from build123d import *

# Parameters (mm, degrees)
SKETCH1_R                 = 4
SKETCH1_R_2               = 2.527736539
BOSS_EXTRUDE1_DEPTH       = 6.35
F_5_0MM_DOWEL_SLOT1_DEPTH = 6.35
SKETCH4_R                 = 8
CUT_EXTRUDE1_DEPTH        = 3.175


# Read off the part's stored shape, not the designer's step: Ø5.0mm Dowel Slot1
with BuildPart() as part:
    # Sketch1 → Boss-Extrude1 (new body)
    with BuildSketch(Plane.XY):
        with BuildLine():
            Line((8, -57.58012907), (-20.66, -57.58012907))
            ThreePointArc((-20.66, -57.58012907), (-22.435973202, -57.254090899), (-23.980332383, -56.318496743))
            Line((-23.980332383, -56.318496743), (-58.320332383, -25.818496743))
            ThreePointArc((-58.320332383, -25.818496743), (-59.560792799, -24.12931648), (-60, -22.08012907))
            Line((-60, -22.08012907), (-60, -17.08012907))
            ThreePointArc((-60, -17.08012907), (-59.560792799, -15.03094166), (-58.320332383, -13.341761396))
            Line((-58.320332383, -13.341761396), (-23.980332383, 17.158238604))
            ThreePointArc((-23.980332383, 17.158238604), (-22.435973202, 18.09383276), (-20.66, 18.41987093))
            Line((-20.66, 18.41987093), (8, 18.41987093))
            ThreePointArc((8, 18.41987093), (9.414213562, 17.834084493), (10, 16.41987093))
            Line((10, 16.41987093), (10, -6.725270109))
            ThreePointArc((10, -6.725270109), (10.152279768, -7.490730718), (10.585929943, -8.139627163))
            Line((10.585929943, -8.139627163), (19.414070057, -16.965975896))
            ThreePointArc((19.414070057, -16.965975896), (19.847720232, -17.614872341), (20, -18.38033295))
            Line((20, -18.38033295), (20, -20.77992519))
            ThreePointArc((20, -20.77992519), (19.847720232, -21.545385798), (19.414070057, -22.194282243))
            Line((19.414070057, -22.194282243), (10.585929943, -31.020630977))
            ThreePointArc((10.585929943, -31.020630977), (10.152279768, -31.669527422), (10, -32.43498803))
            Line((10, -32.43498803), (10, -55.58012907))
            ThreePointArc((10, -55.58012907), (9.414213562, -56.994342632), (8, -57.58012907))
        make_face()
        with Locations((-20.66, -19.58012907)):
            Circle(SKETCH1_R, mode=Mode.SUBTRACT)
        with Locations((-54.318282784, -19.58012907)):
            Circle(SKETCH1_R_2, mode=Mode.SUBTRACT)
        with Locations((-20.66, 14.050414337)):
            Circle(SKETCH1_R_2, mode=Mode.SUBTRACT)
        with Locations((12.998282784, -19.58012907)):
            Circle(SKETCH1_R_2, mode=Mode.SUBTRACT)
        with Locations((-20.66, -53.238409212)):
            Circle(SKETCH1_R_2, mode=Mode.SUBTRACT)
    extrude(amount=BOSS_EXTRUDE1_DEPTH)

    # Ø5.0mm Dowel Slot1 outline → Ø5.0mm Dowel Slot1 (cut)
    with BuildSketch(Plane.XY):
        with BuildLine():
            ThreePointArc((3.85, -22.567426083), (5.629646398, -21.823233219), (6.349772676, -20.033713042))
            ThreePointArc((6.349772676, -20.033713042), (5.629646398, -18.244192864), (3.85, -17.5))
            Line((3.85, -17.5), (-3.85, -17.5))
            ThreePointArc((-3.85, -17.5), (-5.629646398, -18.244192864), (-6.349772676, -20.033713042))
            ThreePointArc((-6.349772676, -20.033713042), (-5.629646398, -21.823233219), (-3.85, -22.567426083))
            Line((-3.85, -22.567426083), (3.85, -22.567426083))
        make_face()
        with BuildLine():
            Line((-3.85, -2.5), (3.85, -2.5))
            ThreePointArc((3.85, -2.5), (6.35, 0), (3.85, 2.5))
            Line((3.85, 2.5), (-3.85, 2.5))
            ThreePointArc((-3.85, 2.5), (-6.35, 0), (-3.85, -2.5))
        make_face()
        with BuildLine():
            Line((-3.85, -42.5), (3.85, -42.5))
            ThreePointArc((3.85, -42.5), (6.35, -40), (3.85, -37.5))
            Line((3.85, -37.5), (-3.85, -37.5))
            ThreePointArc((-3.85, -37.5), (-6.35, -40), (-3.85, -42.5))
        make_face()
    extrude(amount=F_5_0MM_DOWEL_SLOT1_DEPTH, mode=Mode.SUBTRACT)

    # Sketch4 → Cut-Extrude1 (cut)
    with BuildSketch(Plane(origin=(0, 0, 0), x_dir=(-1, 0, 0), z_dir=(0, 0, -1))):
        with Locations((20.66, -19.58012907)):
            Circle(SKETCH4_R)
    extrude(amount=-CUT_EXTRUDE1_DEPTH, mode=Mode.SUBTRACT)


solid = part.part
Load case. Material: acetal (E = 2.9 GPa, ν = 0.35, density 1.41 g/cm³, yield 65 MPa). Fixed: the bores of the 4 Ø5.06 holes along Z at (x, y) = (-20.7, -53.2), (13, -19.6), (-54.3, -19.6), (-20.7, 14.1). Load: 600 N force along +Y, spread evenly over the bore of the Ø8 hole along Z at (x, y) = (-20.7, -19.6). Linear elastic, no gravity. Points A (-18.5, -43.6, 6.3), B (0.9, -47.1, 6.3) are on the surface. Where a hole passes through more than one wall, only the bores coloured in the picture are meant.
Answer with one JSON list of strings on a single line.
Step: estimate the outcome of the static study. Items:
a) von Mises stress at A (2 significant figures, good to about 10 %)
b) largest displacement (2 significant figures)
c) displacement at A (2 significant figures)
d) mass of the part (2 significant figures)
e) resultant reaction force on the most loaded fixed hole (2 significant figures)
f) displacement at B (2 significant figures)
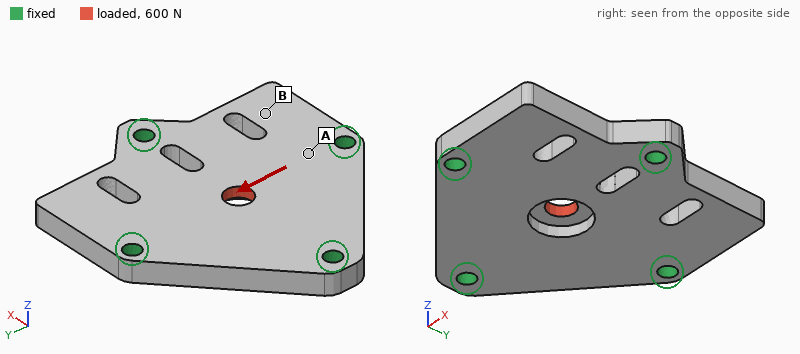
["2.8 MPa", "38 µm", "7.5 µm", "34 g", "230 N", "9.3 µm"]
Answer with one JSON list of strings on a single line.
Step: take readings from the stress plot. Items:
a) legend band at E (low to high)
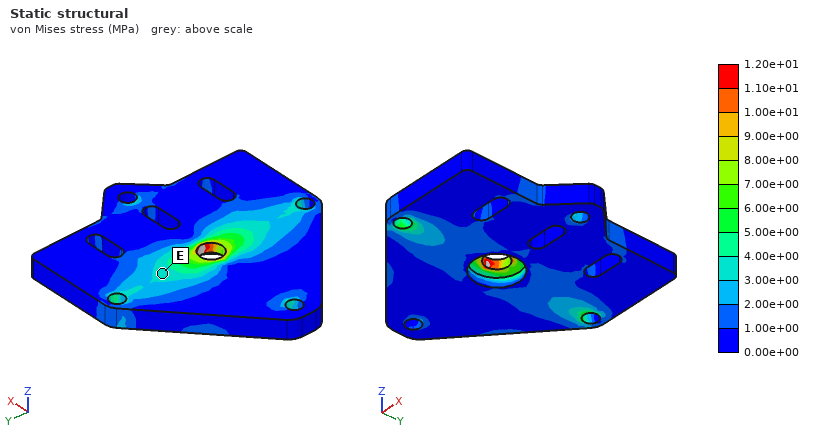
["3.00e+00 to 4.00e+00 MPa"]
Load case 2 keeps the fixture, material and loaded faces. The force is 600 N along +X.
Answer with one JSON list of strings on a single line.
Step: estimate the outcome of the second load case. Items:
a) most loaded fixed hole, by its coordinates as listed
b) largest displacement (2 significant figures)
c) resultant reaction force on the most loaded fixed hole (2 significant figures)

["(-54.3, -19.6)", "43 µm", "250 N"]
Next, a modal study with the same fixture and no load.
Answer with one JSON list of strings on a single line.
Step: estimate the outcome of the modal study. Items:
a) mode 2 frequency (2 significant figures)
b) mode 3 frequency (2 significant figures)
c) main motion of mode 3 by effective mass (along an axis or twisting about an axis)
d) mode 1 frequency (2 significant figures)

["2400 Hz", "2700 Hz", "along Z", "2400 Hz"]
